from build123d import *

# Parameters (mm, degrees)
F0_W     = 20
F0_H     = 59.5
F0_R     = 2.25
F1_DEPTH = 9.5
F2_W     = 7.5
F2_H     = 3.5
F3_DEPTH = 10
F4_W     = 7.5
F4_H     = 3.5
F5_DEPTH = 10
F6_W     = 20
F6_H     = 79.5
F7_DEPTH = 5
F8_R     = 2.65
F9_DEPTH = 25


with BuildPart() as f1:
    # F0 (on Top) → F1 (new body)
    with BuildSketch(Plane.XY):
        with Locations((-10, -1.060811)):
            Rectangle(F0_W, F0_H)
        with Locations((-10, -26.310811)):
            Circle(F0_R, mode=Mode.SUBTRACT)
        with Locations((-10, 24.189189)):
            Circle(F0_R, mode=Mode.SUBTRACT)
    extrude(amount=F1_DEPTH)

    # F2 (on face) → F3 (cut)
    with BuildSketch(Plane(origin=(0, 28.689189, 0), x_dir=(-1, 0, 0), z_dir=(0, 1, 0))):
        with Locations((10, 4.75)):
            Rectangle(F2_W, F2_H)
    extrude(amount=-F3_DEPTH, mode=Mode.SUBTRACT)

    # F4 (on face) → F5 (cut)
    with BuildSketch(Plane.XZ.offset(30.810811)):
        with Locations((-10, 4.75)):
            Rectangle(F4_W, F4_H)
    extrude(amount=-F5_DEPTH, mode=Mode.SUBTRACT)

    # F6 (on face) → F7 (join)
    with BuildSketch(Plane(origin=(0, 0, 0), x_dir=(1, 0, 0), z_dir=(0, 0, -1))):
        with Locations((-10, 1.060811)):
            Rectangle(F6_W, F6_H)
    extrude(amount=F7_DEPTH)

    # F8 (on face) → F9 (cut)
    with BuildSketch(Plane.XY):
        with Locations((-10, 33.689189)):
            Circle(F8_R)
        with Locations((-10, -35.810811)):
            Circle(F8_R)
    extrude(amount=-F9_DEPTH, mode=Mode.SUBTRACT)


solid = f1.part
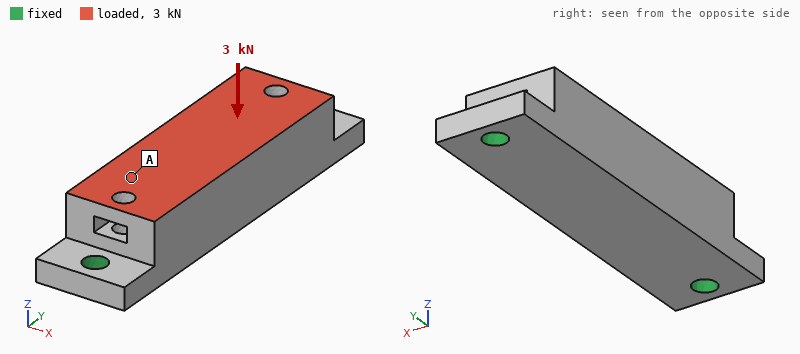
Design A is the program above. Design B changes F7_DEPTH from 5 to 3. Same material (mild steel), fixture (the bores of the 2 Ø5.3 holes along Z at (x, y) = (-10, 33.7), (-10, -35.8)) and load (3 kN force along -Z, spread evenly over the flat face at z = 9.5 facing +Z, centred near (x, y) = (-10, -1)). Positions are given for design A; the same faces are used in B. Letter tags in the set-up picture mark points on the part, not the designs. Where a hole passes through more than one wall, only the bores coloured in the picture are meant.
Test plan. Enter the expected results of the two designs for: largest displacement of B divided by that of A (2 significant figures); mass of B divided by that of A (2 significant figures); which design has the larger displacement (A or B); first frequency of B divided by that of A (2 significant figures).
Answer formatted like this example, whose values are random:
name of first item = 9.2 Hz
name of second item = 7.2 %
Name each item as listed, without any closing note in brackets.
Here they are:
largest displacement of B divided by that of A = 1.7
mass of B divided by that of A = 0.83
which design has the larger displacement = B
first frequency of B divided by that of A = 0.71
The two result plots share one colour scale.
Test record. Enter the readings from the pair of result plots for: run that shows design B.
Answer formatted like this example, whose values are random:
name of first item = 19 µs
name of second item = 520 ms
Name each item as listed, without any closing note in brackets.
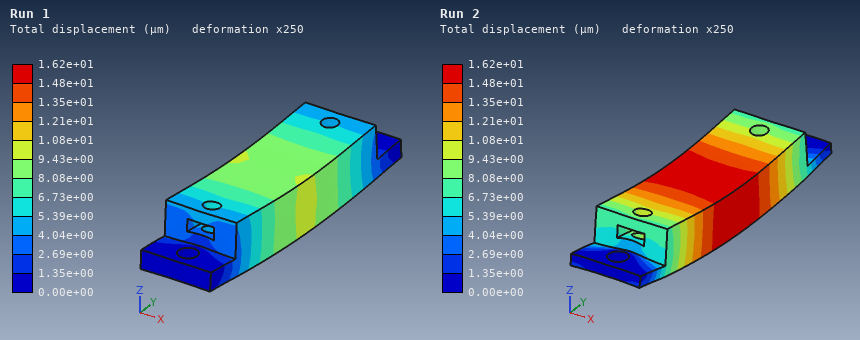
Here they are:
run that shows design B = Run 2
